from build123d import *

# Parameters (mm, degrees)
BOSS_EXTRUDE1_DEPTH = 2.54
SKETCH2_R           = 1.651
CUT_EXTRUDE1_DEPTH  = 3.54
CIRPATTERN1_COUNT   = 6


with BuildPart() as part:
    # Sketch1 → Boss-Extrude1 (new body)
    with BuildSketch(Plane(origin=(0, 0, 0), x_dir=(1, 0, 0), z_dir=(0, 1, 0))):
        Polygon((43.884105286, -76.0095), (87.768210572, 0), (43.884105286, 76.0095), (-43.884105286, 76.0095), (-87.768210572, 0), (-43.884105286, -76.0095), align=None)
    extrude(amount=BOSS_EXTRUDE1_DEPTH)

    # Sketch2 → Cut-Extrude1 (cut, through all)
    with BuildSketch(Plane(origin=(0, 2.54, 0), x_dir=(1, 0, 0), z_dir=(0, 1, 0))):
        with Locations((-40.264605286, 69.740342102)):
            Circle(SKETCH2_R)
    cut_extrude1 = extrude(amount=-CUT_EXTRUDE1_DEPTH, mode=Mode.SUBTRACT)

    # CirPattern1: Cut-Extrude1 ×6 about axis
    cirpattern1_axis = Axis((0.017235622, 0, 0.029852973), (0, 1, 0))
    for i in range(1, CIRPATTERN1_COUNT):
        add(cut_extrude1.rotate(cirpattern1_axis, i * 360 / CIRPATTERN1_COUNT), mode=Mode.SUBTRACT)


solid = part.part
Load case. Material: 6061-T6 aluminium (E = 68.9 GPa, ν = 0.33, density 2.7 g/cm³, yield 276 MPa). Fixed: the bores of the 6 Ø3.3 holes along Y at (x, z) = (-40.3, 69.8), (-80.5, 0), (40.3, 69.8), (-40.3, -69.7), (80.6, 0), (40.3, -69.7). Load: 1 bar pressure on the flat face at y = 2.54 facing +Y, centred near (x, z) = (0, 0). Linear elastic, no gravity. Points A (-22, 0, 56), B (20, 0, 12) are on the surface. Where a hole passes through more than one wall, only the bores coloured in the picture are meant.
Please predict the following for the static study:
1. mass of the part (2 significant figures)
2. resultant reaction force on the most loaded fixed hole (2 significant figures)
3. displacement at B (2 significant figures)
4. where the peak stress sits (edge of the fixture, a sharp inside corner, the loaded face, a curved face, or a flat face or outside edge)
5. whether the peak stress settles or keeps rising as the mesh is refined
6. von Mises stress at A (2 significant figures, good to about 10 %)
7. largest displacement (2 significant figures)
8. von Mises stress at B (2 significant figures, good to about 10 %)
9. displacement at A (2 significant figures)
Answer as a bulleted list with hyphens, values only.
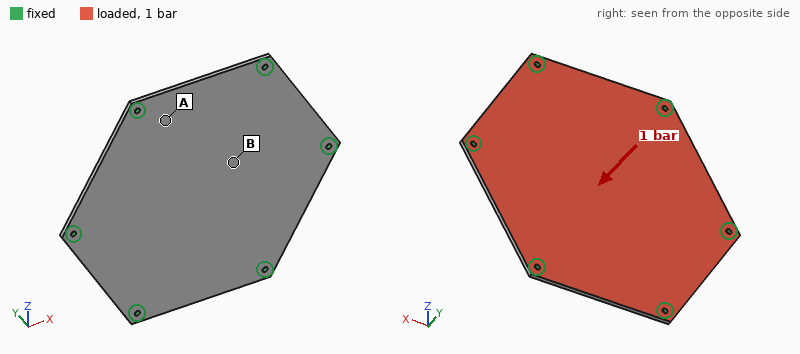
- 140 g
- 330 N
- 0.95 mm
- edge of the fixture
- keeps rising
- 24 MPa
- 1.1 mm
- 60 MPa
- 0.32 mm
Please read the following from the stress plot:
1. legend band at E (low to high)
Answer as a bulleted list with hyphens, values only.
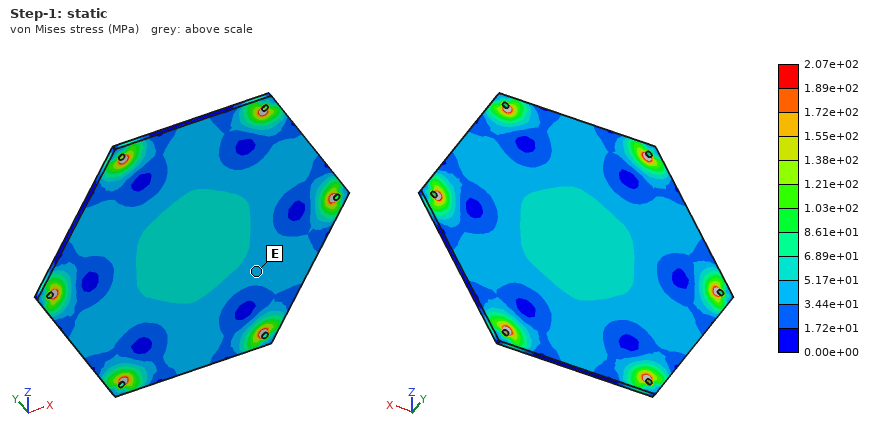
- 3.44e+01 to 5.17e+01 MPa
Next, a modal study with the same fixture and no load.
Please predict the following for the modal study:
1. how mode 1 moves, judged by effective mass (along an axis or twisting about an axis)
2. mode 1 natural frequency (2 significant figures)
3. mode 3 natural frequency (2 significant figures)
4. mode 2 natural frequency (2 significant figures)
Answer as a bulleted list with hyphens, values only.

- along Y
- 730 Hz
- 1500 Hz
- 1500 Hz
